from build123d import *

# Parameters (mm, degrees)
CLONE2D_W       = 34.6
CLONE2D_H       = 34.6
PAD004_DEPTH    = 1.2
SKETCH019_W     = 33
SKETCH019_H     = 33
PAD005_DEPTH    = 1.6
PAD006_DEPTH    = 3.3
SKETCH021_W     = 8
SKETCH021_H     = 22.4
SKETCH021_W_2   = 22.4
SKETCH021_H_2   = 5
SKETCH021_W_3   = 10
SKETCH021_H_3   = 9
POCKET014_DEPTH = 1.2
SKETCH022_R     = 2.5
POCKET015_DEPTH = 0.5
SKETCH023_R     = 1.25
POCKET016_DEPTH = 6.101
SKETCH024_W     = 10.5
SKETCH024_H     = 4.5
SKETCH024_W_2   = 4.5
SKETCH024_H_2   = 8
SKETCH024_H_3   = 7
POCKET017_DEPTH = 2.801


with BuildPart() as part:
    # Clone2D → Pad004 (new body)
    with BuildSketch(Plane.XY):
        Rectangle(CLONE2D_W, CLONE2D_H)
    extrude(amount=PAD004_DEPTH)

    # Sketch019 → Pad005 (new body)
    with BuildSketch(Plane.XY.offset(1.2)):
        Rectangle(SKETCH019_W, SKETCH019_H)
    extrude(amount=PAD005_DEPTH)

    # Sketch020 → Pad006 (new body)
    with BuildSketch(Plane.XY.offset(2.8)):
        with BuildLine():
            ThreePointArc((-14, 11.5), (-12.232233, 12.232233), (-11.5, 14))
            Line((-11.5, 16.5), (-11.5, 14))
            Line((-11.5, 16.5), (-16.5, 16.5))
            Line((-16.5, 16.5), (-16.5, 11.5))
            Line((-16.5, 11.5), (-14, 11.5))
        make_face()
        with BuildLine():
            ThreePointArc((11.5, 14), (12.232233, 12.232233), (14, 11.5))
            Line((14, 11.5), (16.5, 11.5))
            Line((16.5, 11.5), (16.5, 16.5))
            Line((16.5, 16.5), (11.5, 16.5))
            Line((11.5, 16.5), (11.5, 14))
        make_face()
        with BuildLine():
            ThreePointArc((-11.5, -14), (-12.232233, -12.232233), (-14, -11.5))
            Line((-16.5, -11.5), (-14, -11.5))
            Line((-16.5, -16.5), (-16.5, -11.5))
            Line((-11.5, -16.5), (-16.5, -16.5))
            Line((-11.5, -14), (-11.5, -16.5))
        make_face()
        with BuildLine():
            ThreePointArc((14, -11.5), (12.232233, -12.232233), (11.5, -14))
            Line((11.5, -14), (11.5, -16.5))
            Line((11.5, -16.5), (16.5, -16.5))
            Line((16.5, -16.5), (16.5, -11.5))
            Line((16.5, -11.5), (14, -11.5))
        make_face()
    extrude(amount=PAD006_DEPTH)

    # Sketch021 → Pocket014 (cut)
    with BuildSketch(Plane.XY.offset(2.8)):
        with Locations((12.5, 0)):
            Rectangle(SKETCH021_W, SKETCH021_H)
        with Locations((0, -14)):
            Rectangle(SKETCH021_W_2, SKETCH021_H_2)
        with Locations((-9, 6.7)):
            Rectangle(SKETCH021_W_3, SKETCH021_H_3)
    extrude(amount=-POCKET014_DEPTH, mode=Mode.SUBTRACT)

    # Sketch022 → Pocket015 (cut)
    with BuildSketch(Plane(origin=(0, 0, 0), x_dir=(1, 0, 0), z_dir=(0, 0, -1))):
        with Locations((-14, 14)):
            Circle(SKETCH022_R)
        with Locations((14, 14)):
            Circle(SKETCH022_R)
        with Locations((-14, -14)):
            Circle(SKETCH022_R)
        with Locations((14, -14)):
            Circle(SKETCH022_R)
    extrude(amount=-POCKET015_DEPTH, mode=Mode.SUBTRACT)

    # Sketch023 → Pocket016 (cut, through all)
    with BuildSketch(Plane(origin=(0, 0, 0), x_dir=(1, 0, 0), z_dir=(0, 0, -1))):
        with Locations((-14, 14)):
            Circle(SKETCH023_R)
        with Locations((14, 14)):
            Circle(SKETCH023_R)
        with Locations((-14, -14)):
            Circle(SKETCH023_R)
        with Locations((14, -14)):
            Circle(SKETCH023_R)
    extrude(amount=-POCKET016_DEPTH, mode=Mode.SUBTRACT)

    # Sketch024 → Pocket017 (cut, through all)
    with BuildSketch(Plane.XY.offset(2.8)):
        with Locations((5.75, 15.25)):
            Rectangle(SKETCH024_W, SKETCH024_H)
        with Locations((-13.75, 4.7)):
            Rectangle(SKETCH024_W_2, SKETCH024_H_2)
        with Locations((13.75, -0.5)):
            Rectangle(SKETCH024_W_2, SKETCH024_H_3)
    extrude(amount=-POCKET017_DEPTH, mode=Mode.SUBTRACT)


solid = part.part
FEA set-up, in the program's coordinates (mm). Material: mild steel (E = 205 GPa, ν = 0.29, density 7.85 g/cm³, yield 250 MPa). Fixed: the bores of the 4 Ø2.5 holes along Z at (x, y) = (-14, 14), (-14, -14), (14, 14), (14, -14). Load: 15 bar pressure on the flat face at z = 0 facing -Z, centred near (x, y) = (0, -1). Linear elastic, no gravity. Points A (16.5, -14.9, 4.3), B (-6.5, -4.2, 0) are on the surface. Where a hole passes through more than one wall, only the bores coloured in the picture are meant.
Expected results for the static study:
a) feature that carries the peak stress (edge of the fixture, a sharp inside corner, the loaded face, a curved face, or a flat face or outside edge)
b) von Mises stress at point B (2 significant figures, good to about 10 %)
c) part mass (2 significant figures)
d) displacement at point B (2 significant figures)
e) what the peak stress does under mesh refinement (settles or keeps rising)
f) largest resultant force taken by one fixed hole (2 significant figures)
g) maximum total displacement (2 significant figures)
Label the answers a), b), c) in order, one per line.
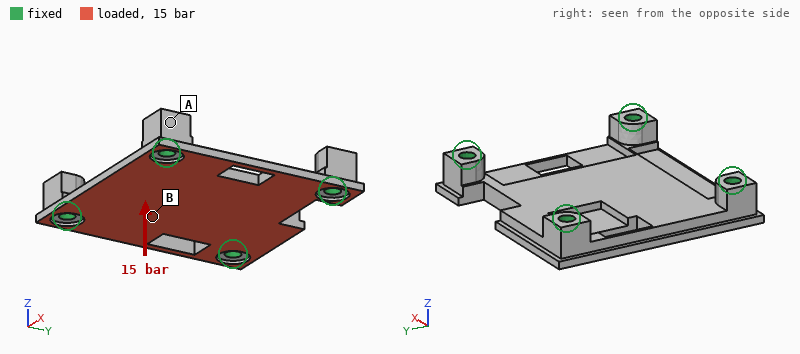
a) a sharp inside corner
b) 43 MPa
c) 21 g
d) 19 µm
e) keeps rising
f) 460 N
g) 25 µm
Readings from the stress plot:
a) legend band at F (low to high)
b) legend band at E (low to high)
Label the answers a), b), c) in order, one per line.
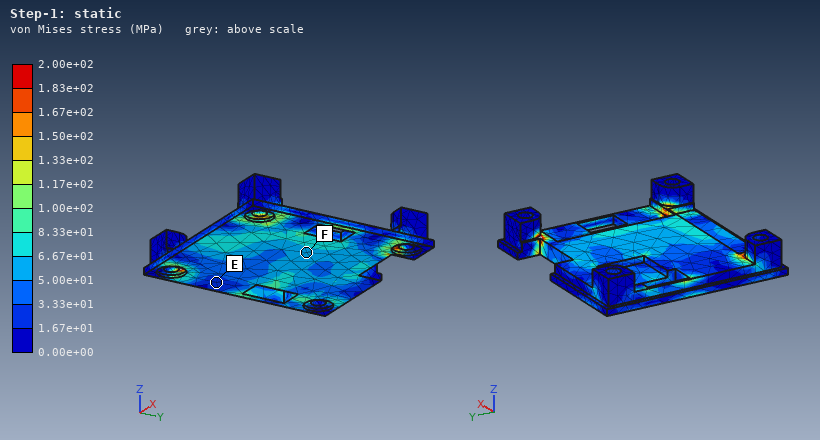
a) 5.00e+01 to 6.67e+01 MPa
b) 1.67e+01 to 3.33e+01 MPa
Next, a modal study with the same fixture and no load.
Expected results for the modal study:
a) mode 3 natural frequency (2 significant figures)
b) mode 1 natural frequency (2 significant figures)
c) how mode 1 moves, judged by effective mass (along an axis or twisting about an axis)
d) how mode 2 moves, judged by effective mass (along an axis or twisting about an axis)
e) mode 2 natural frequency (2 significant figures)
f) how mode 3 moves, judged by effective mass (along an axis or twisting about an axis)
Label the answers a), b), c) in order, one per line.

a) 18 kHz
b) 10 kHz
c) along Z
d) twisting about X
e) 17 kHz
f) twisting about Y
